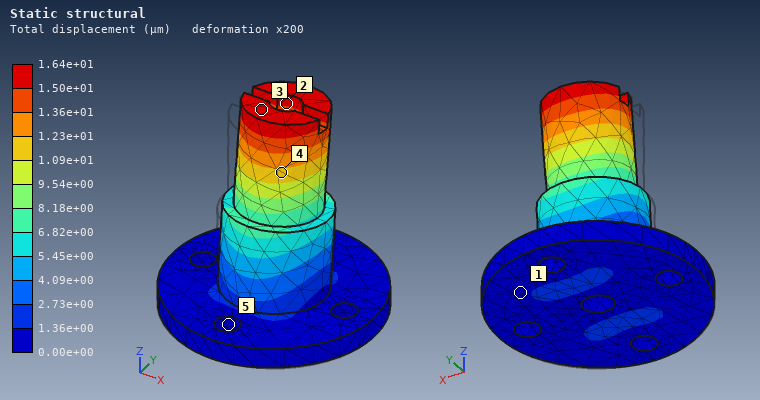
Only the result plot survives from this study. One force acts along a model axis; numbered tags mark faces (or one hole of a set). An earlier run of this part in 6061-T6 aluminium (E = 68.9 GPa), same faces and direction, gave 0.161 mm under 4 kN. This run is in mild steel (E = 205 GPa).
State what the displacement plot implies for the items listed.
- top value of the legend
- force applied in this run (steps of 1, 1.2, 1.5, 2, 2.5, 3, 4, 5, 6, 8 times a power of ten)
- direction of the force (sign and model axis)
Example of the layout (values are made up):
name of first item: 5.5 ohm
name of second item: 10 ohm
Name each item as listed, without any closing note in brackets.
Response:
top value of the legend: 1.64e+01 µm
force applied in this run: 1.2 kN
direction of the force: +Y
